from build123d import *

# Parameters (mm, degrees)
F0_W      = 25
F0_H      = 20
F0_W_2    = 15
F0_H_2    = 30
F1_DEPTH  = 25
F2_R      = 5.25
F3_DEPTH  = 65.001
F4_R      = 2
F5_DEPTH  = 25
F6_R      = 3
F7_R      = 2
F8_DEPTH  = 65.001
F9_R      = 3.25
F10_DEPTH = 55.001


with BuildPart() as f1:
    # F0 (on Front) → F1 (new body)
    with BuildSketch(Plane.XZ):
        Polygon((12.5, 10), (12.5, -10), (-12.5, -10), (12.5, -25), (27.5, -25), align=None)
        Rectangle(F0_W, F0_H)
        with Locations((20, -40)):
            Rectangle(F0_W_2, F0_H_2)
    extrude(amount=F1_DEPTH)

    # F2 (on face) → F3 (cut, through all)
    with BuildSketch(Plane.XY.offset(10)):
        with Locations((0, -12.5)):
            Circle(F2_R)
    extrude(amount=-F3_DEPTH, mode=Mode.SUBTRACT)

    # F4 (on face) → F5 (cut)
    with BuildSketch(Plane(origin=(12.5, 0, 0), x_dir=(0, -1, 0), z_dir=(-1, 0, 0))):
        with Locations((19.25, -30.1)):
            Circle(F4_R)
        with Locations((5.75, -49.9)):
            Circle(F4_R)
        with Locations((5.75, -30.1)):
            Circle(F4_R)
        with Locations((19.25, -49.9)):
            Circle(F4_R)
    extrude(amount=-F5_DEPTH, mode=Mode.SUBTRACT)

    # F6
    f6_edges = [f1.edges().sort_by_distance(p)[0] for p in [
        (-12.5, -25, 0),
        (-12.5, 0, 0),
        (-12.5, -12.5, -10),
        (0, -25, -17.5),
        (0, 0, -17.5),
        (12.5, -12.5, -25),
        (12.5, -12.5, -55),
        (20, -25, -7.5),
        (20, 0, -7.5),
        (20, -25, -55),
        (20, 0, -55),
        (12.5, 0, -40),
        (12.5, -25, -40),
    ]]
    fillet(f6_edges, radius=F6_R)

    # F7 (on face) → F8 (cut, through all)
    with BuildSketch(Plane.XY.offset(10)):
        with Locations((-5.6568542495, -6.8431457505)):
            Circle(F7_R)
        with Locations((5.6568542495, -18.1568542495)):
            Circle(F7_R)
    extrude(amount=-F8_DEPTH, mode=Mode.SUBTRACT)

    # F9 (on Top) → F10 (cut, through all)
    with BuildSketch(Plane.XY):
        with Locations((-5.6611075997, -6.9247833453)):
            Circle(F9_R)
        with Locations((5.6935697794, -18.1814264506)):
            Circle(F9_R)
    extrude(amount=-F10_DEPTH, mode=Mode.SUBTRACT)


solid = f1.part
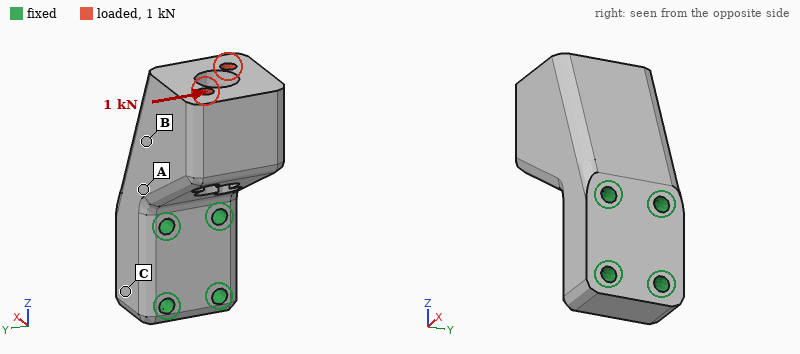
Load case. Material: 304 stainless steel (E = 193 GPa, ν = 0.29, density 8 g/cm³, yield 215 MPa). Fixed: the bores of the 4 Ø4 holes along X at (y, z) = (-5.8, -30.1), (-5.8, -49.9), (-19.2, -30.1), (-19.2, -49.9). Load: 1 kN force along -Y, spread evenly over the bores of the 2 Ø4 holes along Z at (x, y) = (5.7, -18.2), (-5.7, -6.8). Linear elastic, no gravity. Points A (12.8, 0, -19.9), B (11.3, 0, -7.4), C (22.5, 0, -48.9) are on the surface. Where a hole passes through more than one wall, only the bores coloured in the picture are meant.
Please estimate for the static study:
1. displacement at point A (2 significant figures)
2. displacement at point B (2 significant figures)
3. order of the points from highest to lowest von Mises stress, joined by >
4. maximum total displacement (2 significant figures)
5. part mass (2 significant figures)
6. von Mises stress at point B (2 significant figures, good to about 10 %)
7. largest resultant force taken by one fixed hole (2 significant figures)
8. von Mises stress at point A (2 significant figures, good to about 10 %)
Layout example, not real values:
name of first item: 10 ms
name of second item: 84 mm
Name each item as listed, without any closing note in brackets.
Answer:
displacement at point A: 2.4 µm
displacement at point B: 4.7 µm
order of the points from highest to lowest von Mises stress, joined by >: A > B > C
maximum total displacement: 12 µm
part mass: 240 g
von Mises stress at point B: 9.9 MPa
largest resultant force taken by one fixed hole: 2.2 kN
von Mises stress at point A: 18 MPa
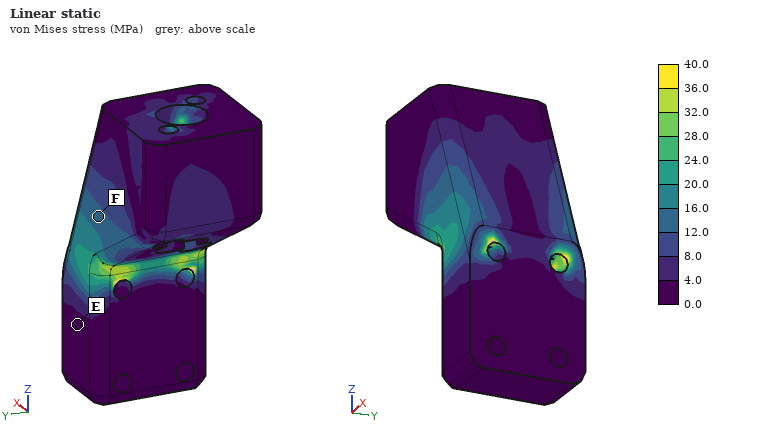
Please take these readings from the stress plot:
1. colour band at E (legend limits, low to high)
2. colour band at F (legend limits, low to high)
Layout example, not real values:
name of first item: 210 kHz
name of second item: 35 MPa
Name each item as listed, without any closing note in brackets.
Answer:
colour band at E: 0.0 to 4.0 MPa
colour band at F: 12.0 to 16.0 MPa
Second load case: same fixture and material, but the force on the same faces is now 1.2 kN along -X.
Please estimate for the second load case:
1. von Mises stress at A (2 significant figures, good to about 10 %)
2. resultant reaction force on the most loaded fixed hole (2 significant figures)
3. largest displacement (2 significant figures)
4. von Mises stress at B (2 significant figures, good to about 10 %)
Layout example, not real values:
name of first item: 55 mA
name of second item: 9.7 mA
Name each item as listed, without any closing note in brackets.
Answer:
von Mises stress at A: 14 MPa
resultant reaction force on the most loaded fixed hole: 720 N
largest displacement: 24 µm
von Mises stress at B: 9.3 MPa
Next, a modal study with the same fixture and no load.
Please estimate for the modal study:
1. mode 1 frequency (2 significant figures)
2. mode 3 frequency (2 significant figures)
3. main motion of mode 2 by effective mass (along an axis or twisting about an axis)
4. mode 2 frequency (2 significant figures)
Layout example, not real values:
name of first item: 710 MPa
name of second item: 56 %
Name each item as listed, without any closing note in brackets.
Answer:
mode 1 frequency: 4300 Hz
mode 3 frequency: 11 kHz
main motion of mode 2 by effective mass: along Y
mode 2 frequency: 5800 Hz
